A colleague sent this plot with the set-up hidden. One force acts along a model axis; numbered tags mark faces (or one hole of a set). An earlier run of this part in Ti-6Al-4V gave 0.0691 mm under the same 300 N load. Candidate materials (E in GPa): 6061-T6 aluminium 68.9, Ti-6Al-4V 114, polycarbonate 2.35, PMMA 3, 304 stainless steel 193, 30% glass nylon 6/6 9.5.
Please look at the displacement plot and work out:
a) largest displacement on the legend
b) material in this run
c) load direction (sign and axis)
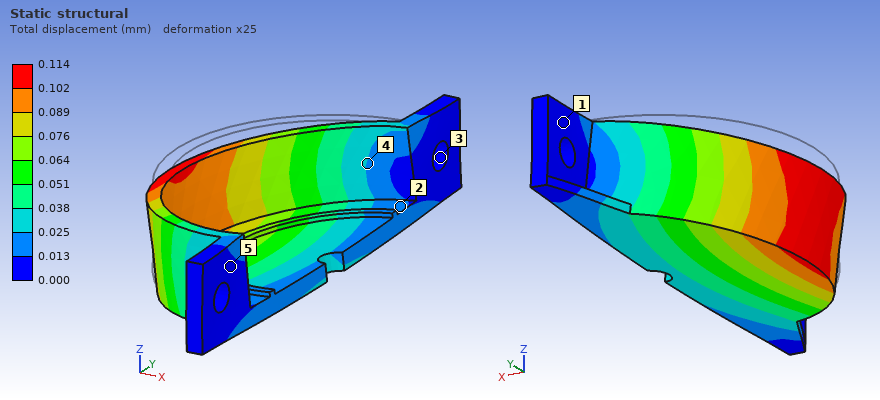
0.114 mm
6061-T6 aluminium
-Z
